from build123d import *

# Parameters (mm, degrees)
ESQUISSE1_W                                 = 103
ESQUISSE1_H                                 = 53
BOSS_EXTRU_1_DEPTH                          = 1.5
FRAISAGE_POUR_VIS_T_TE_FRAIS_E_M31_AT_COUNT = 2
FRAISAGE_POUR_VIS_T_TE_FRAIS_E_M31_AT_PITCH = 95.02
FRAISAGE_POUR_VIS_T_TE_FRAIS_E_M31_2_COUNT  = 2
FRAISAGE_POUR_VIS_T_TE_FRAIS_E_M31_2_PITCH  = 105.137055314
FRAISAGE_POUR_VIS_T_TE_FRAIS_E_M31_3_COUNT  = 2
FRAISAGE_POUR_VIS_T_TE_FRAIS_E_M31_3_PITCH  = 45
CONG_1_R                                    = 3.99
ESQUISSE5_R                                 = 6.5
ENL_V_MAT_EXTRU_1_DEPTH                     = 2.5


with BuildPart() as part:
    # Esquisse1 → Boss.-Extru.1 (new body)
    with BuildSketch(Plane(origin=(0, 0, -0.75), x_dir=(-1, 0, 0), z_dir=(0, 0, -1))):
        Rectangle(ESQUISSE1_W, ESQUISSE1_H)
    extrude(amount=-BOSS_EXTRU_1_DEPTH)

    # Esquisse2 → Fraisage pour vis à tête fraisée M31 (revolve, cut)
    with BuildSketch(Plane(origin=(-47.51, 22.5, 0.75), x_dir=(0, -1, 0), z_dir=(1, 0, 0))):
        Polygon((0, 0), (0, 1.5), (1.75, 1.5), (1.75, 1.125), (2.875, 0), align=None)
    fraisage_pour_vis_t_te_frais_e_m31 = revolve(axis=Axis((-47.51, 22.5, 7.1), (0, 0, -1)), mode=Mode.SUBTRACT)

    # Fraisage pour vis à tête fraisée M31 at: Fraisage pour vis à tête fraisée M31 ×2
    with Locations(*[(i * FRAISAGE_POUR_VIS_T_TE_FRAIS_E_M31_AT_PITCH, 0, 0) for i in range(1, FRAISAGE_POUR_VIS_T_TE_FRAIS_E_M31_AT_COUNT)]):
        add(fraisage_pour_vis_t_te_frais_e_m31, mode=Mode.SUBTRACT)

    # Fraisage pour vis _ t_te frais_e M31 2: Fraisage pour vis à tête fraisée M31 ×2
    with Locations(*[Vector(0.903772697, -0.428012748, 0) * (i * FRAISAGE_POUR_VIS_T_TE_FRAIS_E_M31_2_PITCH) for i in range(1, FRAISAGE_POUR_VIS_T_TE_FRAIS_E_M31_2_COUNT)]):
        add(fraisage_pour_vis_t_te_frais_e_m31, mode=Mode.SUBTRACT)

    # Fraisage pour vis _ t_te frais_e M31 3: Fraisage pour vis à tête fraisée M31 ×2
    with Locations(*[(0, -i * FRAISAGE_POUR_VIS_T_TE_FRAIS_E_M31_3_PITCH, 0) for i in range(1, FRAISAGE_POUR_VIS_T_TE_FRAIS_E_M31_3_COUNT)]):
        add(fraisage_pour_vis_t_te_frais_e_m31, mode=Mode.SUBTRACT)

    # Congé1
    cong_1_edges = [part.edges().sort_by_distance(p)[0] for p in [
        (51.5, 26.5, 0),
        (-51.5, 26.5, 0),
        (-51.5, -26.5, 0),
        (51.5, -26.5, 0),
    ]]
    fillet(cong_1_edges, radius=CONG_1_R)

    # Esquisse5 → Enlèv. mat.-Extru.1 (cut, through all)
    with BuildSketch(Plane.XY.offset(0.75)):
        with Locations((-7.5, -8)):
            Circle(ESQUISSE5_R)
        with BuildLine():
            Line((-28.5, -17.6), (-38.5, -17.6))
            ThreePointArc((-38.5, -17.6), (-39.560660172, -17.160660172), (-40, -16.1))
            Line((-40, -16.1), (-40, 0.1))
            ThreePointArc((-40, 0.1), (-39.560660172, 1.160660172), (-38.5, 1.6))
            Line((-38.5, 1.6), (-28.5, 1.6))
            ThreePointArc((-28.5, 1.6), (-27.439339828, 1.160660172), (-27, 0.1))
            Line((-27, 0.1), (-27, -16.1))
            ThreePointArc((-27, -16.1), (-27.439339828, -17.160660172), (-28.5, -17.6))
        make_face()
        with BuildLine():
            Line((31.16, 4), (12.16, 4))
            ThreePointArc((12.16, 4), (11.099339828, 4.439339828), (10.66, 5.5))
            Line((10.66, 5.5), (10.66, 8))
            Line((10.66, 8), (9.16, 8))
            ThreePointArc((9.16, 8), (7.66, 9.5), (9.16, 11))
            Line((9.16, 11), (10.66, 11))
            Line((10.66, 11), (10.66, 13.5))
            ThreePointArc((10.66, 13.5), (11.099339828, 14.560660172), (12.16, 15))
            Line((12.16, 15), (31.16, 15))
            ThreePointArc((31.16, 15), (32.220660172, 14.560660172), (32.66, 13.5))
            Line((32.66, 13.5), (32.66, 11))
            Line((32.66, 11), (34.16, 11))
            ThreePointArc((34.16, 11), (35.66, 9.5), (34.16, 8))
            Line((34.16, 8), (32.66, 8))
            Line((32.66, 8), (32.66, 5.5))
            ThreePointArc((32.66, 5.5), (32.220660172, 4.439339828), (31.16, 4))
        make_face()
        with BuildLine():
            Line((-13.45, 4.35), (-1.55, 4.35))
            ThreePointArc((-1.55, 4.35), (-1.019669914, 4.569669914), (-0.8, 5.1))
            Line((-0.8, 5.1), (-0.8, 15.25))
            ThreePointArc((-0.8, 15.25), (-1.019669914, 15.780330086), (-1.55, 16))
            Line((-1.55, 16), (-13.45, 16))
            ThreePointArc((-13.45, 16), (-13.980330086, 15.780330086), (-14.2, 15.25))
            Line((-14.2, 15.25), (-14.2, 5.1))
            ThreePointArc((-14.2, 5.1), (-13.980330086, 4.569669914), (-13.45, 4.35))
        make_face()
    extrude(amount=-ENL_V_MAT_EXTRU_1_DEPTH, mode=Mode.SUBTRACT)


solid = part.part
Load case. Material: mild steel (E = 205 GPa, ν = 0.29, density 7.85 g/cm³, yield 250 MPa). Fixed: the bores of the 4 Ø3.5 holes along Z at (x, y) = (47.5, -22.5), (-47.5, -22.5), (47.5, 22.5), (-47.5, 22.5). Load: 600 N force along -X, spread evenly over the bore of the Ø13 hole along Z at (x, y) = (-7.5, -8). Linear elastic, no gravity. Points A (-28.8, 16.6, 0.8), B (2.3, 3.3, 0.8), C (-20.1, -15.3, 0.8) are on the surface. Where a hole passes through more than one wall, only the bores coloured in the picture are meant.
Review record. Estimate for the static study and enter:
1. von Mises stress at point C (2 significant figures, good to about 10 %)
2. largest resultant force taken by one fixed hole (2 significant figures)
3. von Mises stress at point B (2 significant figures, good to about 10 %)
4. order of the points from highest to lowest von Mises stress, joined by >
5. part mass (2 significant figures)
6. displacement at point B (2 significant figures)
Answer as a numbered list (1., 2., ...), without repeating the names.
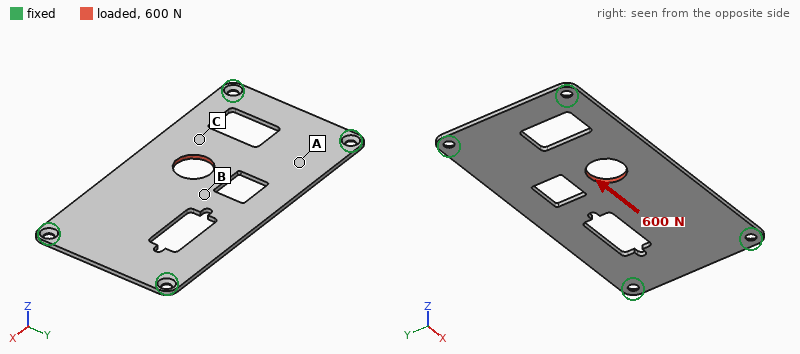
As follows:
1. 11 MPa
2. 190 N
3. 5.9 MPa
4. C > B > A
5. 54 g
6. 2.2 µm
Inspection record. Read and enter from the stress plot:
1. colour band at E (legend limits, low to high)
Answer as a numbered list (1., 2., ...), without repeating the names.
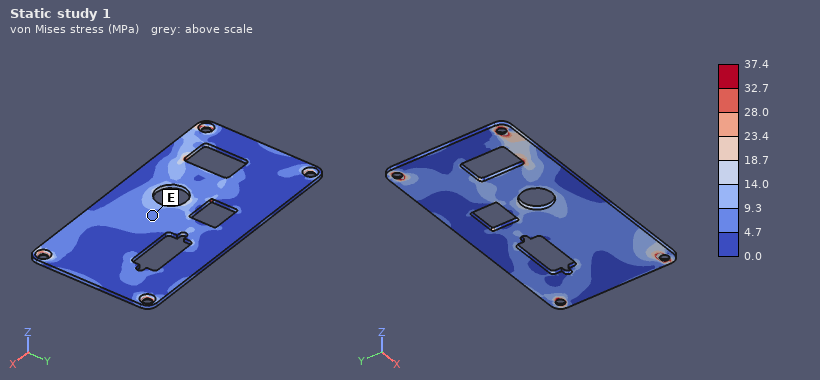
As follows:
1. 4.7 to 9.3 MPa
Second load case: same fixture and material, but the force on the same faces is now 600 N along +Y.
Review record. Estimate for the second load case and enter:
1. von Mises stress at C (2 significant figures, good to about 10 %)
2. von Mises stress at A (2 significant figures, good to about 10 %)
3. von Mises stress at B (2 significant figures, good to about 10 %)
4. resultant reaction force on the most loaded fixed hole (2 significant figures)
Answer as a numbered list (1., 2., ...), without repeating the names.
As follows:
1. 13 MPa
2. 11 MPa
3. 9.8 MPa
4. 240 N
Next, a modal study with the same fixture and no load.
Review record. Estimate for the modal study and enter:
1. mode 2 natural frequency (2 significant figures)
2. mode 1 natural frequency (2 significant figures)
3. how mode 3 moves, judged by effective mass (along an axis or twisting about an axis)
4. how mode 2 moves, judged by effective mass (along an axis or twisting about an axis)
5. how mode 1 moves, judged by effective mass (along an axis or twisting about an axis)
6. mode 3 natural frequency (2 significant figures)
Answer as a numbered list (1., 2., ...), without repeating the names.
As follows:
1. 1200 Hz
2. 690 Hz
3. twisting about Y
4. twisting about X
5. along Z
6. 1900 Hz
